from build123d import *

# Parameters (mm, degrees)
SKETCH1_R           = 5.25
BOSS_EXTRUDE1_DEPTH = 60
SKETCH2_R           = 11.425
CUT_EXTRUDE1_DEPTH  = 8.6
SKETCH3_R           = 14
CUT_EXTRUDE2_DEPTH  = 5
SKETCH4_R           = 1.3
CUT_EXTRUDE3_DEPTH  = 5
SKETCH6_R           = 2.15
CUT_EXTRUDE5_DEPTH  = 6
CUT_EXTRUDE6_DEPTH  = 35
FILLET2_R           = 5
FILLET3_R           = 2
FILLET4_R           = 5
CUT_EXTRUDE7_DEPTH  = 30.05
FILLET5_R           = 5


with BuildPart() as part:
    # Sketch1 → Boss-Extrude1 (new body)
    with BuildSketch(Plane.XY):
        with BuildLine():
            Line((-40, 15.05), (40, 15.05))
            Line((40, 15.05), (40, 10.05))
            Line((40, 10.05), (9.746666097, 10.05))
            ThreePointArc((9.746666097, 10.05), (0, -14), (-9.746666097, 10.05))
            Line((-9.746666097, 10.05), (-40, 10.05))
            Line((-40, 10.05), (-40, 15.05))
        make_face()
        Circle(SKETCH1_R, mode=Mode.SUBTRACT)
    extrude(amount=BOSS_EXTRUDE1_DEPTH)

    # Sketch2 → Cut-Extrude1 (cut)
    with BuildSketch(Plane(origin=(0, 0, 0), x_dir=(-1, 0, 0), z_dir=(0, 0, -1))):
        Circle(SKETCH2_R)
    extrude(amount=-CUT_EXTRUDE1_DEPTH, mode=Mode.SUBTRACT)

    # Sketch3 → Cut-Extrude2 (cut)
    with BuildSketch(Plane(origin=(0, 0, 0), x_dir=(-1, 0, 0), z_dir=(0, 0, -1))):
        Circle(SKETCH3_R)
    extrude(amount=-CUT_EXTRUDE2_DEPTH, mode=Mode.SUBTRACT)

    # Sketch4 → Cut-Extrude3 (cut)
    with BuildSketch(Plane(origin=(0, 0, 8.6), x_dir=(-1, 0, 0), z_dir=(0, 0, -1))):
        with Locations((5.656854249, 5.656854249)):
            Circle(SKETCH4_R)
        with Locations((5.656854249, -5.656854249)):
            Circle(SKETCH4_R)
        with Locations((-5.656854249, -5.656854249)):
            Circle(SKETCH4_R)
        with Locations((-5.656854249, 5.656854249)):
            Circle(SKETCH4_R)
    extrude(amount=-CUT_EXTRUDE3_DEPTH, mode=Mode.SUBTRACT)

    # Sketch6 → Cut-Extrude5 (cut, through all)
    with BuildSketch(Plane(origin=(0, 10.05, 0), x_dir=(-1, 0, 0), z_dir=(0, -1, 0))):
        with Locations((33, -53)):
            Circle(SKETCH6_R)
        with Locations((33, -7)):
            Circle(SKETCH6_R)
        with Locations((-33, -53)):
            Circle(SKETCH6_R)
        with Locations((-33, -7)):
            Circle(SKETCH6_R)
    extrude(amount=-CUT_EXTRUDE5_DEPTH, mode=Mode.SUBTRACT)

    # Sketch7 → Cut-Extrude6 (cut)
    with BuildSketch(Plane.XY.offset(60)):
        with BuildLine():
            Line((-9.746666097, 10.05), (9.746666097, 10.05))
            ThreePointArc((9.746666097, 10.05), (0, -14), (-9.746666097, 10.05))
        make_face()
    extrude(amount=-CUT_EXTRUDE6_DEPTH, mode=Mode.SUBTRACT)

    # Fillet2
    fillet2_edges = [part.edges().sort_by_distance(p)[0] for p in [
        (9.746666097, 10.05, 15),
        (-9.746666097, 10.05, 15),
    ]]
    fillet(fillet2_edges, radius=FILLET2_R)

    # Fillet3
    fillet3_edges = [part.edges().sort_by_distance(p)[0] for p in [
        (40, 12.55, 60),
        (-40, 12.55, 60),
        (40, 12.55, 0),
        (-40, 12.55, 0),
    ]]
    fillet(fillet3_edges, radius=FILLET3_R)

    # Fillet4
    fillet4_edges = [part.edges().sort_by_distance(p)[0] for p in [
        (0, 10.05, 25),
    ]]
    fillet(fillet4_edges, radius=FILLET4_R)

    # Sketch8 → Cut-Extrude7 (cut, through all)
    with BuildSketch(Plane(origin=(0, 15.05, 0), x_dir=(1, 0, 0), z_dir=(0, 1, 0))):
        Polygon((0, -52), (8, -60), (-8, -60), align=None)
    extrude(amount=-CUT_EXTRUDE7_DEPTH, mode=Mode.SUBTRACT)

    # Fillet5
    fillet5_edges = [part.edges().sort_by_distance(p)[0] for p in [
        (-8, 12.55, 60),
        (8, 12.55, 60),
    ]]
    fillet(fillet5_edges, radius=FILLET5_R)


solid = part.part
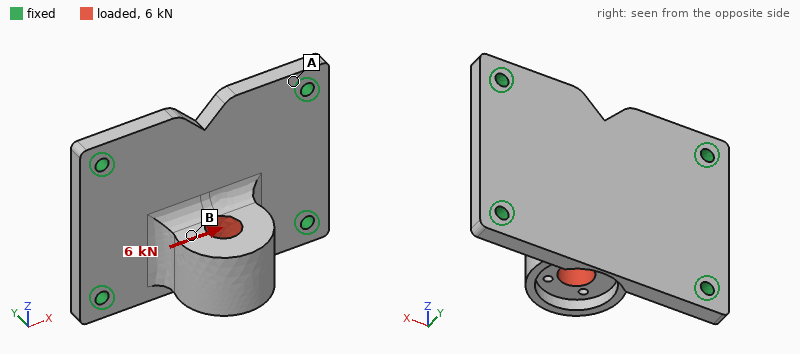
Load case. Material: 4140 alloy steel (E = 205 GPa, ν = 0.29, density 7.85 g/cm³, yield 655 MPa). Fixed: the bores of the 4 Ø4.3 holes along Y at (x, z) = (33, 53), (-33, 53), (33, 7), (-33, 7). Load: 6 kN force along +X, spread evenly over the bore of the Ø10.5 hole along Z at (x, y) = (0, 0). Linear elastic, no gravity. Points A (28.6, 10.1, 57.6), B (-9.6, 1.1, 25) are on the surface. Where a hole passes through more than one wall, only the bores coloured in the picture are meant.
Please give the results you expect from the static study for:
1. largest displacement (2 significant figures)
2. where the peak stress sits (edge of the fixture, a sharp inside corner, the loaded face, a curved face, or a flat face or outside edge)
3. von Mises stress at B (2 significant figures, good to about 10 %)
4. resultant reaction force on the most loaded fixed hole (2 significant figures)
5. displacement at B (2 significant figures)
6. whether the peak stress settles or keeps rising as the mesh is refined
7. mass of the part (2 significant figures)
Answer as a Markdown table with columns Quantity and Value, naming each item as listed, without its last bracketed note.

| Quantity | Value |
|---|---|
| largest displacement | 29 µm |
| where the peak stress sits | edge of the fixture |
| von Mises stress at B | 32 MPa |
| resultant reaction force on the most loaded fixed hole | 2.5 kN |
| displacement at B | 16 µm |
| whether the peak stress settles or keeps rising as the mesh is refined | keeps rising |
| mass of the part | 250 g |
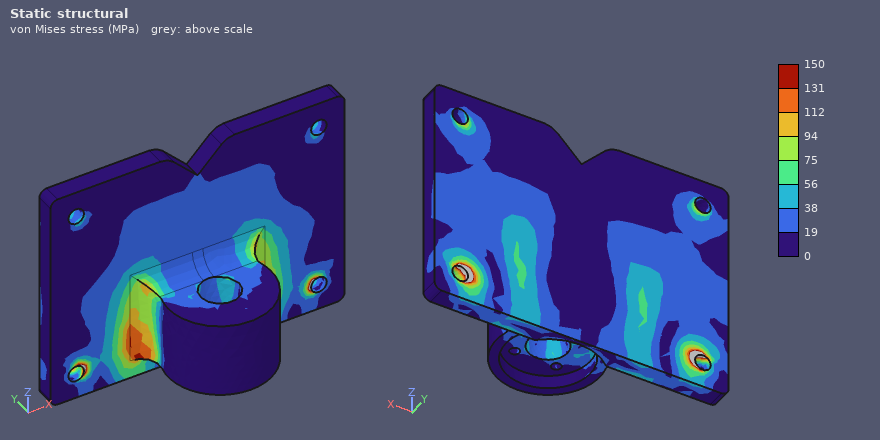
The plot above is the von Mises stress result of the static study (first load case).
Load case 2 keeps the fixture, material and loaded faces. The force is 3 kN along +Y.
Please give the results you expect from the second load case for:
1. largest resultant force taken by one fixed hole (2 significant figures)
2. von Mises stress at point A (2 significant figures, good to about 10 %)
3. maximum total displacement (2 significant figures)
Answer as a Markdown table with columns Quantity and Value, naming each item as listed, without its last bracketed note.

| Quantity | Value |
|---|---|
| largest resultant force taken by one fixed hole | 1.3 kN |
| von Mises stress at point A | 26 MPa |
| maximum total displacement | 27 µm |
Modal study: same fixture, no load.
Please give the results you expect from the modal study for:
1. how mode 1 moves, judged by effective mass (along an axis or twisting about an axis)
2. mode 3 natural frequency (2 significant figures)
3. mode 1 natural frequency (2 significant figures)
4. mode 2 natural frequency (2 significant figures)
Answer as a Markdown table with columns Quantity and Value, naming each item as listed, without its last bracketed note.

| Quantity | Value |
|---|---|
| how mode 1 moves, judged by effective mass | along Y |
| mode 3 natural frequency | 8000 Hz |
| mode 1 natural frequency | 4500 Hz |
| mode 2 natural frequency | 5400 Hz |
